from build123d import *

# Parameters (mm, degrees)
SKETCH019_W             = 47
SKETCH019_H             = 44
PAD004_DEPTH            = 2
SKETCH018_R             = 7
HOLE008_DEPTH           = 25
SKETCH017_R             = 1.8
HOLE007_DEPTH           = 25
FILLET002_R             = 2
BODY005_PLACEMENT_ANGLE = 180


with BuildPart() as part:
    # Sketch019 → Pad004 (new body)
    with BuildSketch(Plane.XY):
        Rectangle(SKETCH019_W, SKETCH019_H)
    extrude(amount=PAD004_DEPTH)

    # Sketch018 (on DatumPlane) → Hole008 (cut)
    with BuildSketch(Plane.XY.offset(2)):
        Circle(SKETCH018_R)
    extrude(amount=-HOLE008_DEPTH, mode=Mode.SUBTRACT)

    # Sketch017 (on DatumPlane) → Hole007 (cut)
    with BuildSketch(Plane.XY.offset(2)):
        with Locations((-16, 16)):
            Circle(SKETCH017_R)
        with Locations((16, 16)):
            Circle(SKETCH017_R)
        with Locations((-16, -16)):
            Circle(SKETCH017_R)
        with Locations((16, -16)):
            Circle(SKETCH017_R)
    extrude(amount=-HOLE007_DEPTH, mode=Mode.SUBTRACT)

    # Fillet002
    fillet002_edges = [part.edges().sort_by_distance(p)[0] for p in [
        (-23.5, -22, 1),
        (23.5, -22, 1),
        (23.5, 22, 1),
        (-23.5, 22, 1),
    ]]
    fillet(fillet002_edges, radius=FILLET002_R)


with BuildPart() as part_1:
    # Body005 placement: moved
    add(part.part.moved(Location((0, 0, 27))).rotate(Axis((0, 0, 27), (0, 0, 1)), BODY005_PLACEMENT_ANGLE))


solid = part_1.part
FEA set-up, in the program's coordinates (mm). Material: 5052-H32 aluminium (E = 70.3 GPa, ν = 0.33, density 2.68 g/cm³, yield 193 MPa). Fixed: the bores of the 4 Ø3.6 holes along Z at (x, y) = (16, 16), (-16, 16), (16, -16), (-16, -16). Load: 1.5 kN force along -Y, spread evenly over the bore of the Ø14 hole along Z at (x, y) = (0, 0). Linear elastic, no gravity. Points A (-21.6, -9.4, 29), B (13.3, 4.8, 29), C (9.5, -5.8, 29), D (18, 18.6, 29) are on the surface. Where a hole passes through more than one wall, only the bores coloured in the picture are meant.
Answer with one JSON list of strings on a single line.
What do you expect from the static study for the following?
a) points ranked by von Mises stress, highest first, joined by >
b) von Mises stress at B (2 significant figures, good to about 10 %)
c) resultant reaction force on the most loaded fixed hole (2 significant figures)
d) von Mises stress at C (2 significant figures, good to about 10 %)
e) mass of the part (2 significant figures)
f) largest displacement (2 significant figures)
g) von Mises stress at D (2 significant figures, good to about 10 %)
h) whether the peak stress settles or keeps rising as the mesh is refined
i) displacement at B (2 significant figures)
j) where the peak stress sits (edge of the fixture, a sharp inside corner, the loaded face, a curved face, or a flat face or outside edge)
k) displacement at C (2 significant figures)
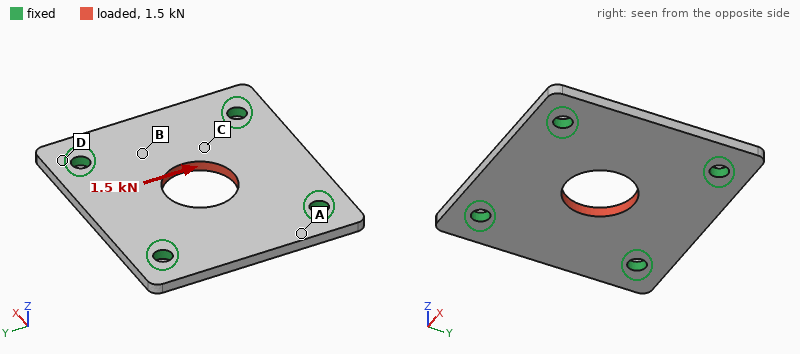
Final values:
["C > B > D > A", "13 MPa", "410 N", "17 MPa", "10 g", "6.1 µm", "8.2 MPa", "keeps rising", "2.1 µm", "edge of the fixture", "3.3 µm"]
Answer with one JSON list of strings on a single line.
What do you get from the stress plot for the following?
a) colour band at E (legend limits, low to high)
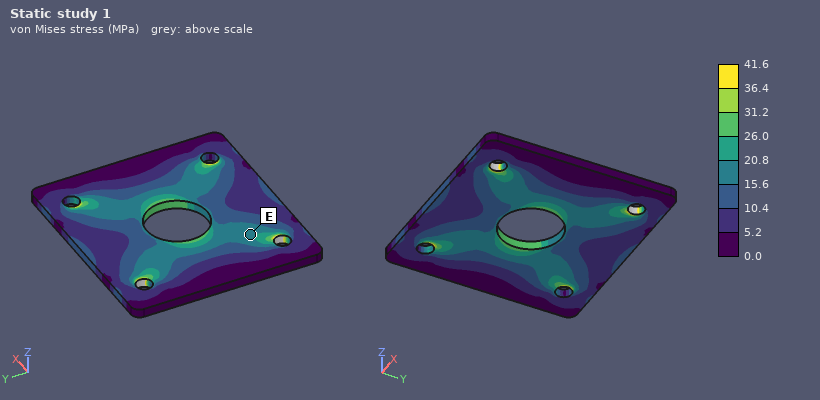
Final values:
["15.6 to 20.8 MPa"]
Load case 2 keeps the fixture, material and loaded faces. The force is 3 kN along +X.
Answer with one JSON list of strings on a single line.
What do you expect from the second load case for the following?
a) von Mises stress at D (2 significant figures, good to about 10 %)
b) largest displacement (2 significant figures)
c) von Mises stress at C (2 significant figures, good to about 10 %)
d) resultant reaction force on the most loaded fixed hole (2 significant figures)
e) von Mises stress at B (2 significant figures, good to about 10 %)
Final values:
["14 MPa", "12 µm", "31 MPa", "800 N", "24 MPa"]
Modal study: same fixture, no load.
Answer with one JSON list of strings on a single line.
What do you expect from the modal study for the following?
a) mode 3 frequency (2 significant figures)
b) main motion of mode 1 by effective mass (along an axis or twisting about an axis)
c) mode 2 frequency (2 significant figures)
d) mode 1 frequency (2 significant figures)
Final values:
["11 kHz", "along Z", "11 kHz", "8600 Hz"]
